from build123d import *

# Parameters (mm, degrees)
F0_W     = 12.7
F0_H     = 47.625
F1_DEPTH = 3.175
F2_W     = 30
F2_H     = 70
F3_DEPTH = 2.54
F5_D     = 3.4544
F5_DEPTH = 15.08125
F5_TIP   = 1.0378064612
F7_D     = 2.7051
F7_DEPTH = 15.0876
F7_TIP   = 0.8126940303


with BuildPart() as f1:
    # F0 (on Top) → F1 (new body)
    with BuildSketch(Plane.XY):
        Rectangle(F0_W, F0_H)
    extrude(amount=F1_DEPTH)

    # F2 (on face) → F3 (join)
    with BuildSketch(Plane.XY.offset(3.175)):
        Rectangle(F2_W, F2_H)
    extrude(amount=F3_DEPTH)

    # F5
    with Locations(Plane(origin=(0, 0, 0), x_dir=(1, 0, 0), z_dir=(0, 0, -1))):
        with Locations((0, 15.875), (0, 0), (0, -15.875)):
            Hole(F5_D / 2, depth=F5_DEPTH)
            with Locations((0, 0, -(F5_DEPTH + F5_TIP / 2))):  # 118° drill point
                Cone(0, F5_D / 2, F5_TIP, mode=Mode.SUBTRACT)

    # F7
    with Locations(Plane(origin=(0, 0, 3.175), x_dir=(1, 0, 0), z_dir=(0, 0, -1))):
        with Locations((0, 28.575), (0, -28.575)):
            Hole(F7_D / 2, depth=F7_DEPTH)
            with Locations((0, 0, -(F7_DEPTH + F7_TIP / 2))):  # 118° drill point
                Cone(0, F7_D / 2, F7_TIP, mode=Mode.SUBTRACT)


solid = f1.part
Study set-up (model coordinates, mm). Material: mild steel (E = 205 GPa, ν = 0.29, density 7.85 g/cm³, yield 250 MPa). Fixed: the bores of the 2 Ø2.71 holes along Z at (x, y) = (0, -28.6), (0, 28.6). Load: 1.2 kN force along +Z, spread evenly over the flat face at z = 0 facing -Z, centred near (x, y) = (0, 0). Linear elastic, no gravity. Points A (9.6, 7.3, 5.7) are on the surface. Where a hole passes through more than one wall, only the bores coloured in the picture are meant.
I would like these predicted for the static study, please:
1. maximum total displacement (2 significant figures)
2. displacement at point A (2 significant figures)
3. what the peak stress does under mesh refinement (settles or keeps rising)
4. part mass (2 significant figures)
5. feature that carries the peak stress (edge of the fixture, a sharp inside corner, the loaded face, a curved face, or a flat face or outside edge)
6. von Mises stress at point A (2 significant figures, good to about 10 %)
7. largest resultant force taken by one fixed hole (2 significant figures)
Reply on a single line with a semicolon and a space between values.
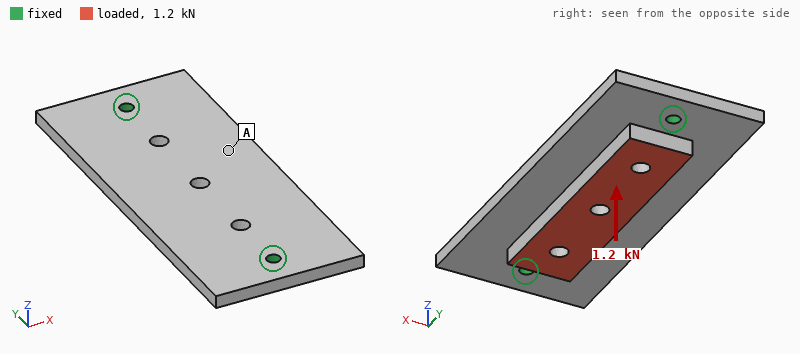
38 µm; 33 µm; keeps rising; 55 g; edge of the fixture; 36 MPa; 980 N
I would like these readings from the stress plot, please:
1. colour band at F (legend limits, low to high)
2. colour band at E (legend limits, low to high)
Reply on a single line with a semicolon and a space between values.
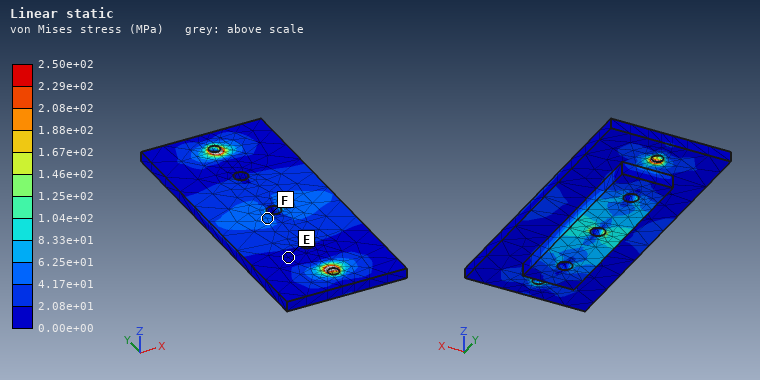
4.17e+01 to 6.25e+01 MPa; 0.00e+00 to 2.08e+01 MPa
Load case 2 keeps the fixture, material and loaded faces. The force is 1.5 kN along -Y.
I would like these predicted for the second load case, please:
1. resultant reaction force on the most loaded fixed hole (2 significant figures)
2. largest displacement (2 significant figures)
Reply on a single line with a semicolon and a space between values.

760 N; 1.6 µm
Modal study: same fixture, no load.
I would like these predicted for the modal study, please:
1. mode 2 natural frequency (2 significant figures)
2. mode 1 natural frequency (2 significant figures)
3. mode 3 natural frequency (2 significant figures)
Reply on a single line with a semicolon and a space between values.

4900 Hz; 4700 Hz; 9900 Hz
